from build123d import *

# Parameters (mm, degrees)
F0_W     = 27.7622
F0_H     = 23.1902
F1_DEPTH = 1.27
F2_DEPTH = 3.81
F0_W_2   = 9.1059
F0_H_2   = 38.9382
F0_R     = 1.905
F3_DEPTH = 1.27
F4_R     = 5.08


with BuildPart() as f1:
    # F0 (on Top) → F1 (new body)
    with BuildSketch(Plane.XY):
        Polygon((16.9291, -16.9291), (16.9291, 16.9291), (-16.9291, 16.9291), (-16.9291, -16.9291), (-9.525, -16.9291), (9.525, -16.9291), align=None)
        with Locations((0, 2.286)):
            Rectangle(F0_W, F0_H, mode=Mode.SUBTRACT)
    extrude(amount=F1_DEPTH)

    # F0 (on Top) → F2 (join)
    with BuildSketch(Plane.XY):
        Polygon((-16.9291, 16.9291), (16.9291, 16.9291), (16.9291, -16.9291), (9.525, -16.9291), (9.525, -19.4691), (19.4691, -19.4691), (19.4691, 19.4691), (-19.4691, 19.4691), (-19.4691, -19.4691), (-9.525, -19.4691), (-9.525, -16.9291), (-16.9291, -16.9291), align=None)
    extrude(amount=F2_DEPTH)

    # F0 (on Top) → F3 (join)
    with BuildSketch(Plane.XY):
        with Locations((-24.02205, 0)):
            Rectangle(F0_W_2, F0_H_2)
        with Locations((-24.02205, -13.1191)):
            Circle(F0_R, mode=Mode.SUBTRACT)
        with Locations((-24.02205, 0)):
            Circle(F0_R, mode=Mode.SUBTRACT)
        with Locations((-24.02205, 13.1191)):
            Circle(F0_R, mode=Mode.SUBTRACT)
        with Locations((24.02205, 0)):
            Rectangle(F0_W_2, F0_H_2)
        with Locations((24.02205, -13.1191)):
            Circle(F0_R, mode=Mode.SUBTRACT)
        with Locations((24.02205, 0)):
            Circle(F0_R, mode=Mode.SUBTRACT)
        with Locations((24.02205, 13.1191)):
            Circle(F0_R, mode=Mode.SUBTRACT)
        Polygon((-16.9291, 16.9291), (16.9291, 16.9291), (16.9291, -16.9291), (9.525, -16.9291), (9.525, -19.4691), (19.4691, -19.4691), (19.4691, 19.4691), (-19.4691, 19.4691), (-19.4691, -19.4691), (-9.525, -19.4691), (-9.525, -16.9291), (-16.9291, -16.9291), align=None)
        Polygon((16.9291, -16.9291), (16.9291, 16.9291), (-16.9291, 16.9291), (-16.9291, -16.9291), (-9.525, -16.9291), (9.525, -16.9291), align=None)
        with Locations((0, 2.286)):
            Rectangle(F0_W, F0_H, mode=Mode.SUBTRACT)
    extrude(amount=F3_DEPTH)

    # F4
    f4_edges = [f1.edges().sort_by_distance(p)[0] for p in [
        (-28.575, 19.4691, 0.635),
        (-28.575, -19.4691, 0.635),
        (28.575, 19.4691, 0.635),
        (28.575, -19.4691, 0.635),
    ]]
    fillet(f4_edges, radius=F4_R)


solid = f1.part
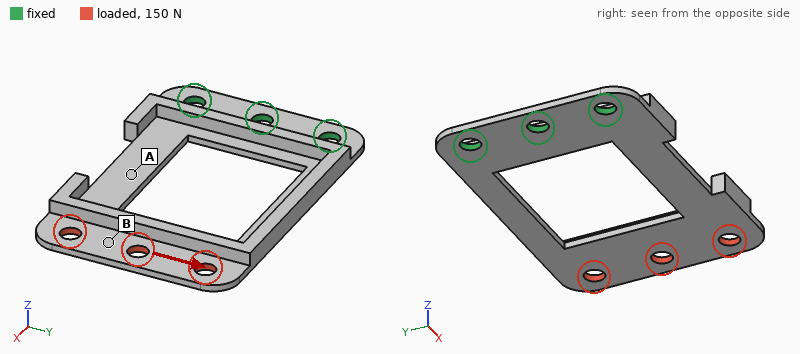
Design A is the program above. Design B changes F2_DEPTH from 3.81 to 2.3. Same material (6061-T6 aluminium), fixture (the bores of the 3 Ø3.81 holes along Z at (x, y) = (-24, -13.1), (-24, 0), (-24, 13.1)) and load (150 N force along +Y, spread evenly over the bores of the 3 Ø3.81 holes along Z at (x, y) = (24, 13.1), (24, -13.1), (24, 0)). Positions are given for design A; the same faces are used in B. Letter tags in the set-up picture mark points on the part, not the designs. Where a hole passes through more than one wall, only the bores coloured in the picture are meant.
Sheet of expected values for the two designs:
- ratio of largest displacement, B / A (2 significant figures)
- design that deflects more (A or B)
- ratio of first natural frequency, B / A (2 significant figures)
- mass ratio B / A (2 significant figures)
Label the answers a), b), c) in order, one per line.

a) 1.1
b) B
c) 0.84
d) 0.82
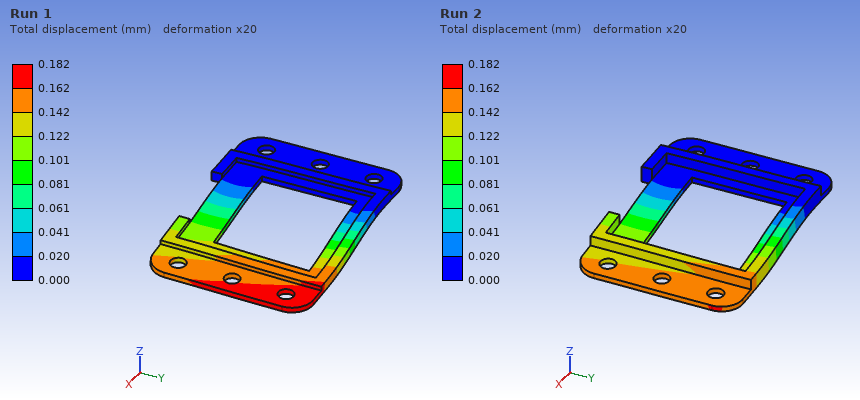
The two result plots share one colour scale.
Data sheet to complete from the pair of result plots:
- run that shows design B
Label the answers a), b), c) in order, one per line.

a) Run 1
